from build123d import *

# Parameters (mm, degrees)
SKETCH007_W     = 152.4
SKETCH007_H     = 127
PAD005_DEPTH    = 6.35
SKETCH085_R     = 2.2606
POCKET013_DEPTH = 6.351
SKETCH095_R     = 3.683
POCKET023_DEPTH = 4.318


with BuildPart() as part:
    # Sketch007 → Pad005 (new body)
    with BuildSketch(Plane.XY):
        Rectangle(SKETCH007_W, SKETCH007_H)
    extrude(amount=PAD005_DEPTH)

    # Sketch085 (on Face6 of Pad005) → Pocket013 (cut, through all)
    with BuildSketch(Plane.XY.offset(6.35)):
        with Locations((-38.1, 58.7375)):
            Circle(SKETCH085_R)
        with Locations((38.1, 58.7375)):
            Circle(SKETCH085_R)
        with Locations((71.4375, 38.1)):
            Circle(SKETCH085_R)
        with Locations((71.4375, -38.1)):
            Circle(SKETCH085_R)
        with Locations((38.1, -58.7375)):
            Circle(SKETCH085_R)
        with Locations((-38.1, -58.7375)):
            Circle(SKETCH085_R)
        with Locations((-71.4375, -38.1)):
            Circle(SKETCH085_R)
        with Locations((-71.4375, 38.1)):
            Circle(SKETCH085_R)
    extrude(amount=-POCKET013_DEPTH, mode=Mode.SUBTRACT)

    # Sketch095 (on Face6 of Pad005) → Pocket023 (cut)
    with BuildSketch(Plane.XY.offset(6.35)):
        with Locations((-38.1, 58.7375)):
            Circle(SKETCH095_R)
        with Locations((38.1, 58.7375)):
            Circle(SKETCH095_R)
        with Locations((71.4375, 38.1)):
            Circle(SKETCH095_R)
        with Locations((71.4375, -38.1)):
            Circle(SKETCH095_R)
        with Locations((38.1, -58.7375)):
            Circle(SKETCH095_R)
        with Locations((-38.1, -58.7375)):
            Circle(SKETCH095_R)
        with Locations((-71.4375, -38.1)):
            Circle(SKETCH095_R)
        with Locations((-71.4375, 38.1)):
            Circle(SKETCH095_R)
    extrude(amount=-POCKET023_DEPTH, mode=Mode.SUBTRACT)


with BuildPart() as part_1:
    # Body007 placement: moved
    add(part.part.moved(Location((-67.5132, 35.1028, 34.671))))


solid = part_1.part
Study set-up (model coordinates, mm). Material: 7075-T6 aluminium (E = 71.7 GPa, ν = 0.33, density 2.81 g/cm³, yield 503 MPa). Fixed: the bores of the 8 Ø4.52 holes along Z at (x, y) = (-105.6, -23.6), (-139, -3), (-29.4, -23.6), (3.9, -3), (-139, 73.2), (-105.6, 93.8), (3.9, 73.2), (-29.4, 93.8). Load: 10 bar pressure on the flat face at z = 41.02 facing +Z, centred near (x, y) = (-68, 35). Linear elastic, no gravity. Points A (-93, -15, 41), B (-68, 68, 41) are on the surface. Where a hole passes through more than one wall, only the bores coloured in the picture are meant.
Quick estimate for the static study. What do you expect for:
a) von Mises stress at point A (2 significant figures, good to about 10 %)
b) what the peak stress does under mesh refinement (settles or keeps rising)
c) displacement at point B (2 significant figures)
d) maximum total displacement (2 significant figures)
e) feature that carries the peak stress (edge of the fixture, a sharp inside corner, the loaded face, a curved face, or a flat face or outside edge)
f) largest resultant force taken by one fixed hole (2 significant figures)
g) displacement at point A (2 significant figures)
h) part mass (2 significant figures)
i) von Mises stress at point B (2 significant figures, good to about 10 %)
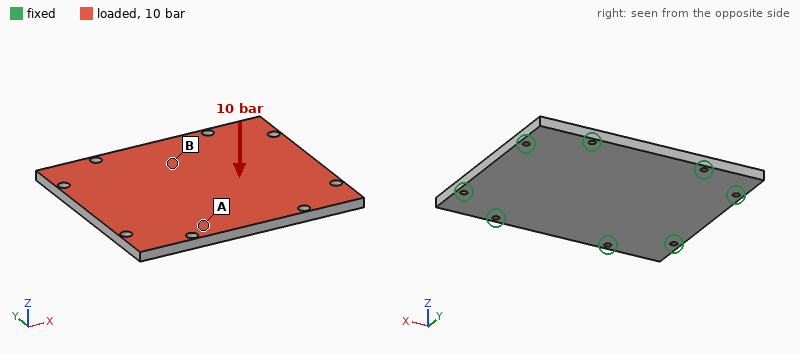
43 MPa
keeps rising
0.45 mm
0.62 mm
edge of the fixture
5.7 kN
0.18 mm
340 g
91 MPa
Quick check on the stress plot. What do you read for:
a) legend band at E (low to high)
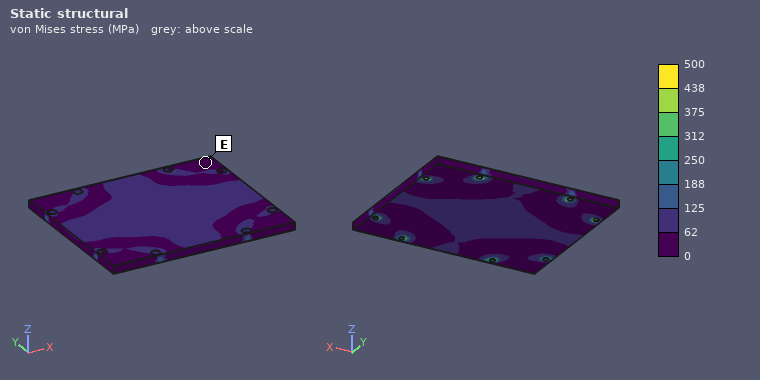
0 to 62 MPa
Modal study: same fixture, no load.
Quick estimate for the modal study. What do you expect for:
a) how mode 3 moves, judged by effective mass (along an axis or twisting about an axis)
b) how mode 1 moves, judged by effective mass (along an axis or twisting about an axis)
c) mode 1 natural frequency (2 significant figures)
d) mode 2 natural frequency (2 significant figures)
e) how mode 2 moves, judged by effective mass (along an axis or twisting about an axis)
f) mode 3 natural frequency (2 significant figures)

twisting about X
along Z
1800 Hz
3400 Hz
twisting about Y
3900 Hz
